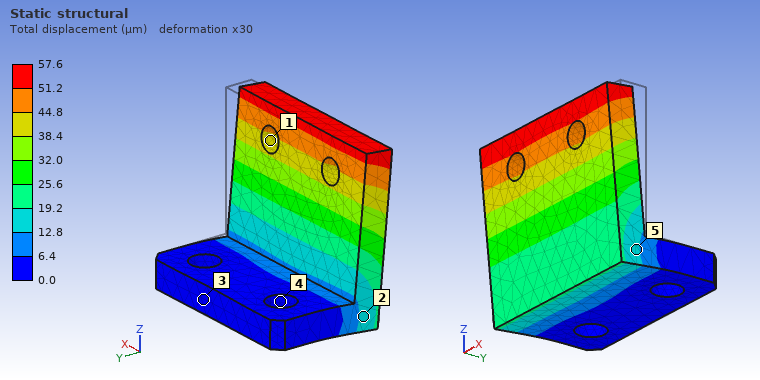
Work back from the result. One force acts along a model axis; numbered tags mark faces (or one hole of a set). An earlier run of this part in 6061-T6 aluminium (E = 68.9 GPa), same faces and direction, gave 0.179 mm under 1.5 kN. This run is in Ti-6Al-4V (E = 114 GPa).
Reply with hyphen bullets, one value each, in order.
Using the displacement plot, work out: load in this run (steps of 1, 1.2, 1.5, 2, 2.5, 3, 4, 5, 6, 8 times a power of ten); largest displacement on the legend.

- 800 N
- 57.6 µm
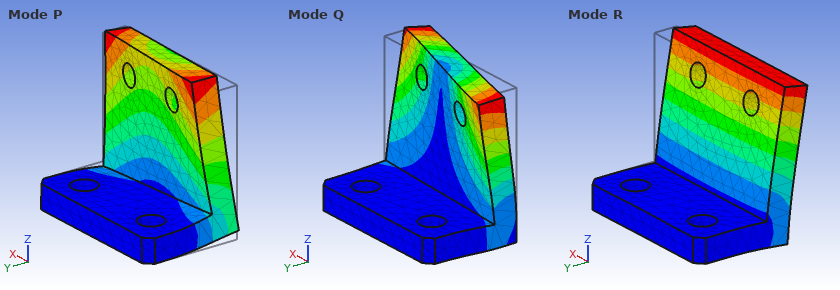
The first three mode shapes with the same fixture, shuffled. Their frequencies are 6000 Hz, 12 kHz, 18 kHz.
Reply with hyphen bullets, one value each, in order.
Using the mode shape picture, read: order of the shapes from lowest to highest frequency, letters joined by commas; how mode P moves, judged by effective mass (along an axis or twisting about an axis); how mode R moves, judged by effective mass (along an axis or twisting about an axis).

- R, P, Q
- along X
- along Y
